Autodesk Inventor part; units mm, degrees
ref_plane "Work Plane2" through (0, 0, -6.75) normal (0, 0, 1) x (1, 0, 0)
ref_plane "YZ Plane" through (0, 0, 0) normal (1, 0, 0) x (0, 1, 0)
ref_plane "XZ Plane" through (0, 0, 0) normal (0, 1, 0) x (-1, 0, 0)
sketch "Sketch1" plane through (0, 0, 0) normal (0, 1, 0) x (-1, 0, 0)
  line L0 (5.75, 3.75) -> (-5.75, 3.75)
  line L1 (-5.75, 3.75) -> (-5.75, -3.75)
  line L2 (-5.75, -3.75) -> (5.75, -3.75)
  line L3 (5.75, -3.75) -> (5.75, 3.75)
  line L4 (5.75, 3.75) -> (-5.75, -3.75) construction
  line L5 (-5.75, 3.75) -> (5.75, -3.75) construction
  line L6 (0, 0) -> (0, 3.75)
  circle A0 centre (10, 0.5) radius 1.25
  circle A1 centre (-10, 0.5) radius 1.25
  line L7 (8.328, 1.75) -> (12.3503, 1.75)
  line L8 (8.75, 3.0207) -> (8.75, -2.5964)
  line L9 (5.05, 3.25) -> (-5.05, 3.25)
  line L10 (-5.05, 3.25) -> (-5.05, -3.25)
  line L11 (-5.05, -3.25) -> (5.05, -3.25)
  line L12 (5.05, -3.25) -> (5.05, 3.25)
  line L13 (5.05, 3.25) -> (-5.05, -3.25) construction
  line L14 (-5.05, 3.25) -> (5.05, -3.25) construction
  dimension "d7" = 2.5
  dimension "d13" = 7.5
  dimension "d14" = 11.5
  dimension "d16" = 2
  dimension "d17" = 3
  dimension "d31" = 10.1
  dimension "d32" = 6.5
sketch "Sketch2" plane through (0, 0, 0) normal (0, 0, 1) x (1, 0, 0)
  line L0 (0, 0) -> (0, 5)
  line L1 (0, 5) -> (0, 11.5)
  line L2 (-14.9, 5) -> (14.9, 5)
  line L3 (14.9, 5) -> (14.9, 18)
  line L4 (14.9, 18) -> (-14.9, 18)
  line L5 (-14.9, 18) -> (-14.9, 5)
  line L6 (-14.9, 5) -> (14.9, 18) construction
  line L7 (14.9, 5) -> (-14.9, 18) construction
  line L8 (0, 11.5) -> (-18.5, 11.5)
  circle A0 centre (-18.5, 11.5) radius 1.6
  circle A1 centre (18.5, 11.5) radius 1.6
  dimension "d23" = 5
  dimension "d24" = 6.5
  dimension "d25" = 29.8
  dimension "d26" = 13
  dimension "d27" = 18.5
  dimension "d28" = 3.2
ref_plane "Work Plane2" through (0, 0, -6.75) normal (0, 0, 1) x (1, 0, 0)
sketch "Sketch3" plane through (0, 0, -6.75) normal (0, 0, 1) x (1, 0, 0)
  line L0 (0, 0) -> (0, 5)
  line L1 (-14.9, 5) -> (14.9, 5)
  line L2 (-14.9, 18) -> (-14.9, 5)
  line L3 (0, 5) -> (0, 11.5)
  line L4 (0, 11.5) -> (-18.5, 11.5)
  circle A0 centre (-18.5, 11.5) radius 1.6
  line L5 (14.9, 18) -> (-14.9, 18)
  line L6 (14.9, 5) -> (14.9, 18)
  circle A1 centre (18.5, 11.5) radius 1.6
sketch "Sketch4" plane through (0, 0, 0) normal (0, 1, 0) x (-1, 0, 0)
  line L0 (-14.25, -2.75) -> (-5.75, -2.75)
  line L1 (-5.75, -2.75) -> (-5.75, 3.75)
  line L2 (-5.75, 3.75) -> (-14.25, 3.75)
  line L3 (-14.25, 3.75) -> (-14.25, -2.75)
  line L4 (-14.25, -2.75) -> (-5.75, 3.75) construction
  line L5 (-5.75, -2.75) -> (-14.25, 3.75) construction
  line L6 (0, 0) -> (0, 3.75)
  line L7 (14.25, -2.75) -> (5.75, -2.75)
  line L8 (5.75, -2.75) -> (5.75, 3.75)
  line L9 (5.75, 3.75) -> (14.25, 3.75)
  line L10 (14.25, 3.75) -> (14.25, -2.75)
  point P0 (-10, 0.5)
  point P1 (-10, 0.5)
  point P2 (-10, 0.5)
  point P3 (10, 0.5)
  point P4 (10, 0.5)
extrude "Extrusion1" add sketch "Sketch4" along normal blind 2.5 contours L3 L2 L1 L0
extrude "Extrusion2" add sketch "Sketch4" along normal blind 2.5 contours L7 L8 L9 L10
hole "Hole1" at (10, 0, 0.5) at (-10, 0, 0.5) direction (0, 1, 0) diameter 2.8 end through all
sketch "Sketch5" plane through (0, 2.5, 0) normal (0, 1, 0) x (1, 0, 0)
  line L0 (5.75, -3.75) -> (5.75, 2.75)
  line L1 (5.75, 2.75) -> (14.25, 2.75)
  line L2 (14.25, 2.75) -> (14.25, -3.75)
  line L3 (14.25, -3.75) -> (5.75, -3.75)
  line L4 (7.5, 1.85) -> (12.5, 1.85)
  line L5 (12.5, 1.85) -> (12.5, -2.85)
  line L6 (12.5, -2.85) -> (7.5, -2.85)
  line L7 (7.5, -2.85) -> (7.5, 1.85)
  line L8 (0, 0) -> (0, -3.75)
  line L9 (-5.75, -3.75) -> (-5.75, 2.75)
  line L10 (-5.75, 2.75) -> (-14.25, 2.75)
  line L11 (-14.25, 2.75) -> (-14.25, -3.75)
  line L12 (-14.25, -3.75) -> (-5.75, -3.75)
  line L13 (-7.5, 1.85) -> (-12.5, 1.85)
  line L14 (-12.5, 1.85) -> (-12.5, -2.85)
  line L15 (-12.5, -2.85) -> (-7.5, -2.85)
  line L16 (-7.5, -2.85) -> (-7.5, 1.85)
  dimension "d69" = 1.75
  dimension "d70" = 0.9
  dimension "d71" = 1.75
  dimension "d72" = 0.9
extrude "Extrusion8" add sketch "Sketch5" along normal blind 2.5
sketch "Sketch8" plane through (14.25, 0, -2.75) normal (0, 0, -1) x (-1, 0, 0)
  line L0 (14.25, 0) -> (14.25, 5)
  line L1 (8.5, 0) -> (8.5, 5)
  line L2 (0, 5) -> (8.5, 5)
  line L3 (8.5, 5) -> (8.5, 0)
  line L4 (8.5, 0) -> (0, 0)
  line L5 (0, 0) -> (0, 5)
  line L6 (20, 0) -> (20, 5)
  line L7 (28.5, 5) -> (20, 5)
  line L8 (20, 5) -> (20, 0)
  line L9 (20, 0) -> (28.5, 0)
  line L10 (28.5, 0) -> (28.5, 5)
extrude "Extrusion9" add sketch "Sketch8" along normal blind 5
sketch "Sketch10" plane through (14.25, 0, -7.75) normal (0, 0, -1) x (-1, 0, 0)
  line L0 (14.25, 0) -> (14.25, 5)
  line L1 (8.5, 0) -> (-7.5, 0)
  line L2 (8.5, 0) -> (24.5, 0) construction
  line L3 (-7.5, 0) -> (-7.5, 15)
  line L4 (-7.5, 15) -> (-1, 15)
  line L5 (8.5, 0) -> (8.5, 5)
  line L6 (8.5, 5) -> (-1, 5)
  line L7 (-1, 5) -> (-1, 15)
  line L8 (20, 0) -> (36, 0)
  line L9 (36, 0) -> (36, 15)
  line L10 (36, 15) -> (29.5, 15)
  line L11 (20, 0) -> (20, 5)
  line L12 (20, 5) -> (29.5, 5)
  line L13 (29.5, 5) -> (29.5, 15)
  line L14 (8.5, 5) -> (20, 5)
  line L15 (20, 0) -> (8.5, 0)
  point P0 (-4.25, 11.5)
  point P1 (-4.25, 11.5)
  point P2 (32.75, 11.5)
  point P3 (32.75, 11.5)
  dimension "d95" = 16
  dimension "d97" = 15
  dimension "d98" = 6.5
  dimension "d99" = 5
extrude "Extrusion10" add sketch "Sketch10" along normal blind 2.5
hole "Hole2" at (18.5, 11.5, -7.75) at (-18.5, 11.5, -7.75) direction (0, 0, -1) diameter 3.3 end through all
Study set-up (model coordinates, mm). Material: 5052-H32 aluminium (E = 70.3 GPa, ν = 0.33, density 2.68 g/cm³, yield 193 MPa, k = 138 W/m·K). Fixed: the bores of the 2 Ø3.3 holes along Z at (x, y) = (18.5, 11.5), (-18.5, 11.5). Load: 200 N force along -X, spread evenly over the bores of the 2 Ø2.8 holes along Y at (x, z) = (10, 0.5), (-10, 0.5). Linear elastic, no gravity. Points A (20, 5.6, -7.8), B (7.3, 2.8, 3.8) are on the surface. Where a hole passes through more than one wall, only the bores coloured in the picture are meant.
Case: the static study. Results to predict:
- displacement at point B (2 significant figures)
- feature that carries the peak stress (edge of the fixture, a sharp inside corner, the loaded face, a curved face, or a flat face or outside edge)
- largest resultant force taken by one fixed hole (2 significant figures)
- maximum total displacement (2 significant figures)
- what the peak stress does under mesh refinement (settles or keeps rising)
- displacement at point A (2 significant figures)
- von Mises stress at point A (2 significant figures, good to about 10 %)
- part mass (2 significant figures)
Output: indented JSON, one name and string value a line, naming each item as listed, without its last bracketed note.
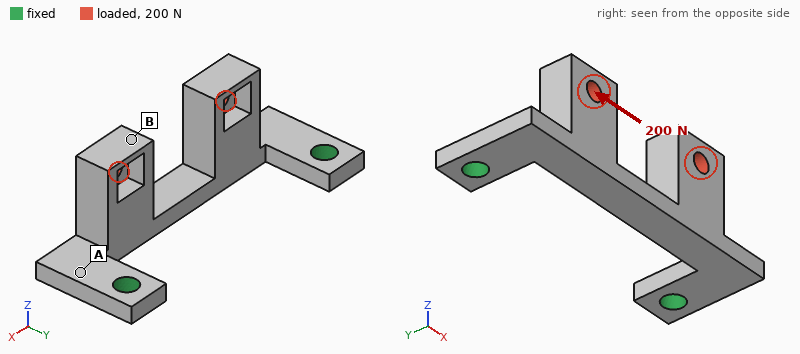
{
  "displacement at point B": "35 µm",
  "feature that carries the peak stress": "edge of the fixture",
  "largest resultant force taken by one fixed hole": "110 N",
  "maximum total displacement": "38 µm",
  "what the peak stress does under mesh refinement": "keeps rising",
  "displacement at point A": "6.1 µm",
  "von Mises stress at point A": "16 MPa",
  "part mass": "4.4 g"
}
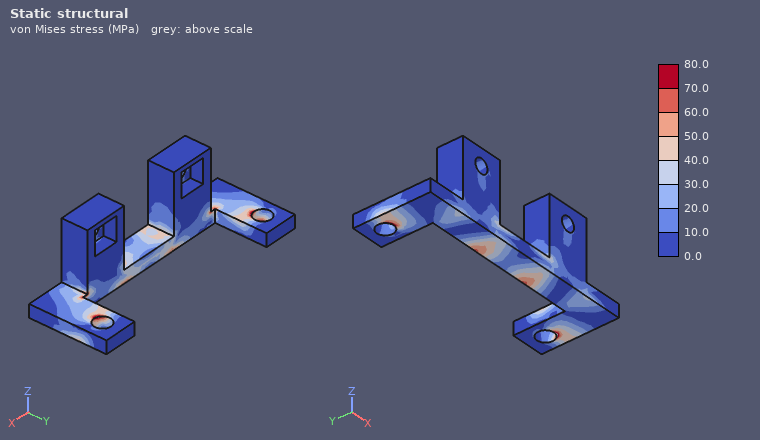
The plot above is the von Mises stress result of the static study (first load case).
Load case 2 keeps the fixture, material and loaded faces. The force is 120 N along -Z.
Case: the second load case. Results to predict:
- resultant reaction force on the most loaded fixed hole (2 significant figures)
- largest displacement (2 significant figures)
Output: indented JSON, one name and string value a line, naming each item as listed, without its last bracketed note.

{
  "resultant reaction force on the most loaded fixed hole": "60 N",
  "largest displacement": "0.11 mm"
}
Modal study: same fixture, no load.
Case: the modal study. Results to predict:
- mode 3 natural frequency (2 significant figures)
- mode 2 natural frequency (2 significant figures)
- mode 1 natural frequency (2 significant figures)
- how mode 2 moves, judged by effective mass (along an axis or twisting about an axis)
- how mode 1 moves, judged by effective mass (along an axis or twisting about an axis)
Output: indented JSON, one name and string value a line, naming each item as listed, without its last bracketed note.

{
  "mode 3 natural frequency": "6300 Hz",
  "mode 2 natural frequency": "5000 Hz",
  "mode 1 natural frequency": "3400 Hz",
  "how mode 2 moves, judged by effective mass": "along Y",
  "how mode 1 moves, judged by effective mass": "along Z"
}
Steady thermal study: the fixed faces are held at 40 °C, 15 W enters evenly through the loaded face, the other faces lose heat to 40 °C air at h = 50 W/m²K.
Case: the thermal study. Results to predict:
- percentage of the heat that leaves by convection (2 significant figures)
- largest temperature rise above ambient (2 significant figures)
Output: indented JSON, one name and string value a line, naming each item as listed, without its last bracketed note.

{
  "percentage of the heat that leaves by convection": "18 %",
  "largest temperature rise above ambient": "52 K"
}
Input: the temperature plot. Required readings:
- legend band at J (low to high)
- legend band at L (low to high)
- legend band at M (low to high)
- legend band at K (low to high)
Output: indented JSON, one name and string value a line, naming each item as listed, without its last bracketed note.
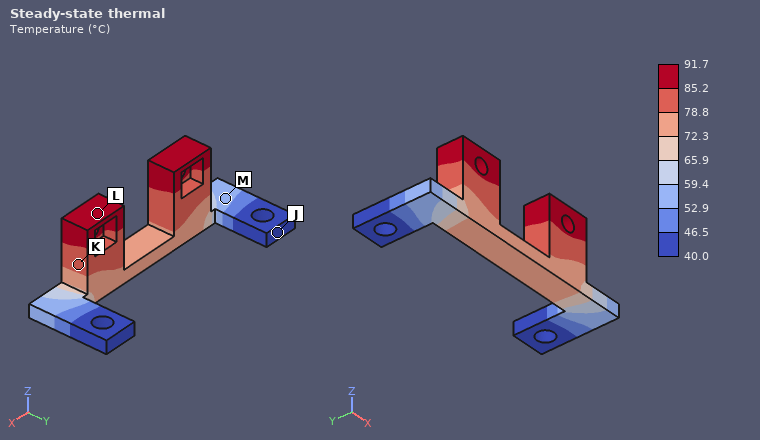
{
  "legend band at J": "40.0 to 46.5 °C",
  "legend band at L": "85.2 to 91.7 °C",
  "legend band at M": "52.9 to 59.4 °C",
  "legend band at K": "78.8 to 85.2 °C"
}
